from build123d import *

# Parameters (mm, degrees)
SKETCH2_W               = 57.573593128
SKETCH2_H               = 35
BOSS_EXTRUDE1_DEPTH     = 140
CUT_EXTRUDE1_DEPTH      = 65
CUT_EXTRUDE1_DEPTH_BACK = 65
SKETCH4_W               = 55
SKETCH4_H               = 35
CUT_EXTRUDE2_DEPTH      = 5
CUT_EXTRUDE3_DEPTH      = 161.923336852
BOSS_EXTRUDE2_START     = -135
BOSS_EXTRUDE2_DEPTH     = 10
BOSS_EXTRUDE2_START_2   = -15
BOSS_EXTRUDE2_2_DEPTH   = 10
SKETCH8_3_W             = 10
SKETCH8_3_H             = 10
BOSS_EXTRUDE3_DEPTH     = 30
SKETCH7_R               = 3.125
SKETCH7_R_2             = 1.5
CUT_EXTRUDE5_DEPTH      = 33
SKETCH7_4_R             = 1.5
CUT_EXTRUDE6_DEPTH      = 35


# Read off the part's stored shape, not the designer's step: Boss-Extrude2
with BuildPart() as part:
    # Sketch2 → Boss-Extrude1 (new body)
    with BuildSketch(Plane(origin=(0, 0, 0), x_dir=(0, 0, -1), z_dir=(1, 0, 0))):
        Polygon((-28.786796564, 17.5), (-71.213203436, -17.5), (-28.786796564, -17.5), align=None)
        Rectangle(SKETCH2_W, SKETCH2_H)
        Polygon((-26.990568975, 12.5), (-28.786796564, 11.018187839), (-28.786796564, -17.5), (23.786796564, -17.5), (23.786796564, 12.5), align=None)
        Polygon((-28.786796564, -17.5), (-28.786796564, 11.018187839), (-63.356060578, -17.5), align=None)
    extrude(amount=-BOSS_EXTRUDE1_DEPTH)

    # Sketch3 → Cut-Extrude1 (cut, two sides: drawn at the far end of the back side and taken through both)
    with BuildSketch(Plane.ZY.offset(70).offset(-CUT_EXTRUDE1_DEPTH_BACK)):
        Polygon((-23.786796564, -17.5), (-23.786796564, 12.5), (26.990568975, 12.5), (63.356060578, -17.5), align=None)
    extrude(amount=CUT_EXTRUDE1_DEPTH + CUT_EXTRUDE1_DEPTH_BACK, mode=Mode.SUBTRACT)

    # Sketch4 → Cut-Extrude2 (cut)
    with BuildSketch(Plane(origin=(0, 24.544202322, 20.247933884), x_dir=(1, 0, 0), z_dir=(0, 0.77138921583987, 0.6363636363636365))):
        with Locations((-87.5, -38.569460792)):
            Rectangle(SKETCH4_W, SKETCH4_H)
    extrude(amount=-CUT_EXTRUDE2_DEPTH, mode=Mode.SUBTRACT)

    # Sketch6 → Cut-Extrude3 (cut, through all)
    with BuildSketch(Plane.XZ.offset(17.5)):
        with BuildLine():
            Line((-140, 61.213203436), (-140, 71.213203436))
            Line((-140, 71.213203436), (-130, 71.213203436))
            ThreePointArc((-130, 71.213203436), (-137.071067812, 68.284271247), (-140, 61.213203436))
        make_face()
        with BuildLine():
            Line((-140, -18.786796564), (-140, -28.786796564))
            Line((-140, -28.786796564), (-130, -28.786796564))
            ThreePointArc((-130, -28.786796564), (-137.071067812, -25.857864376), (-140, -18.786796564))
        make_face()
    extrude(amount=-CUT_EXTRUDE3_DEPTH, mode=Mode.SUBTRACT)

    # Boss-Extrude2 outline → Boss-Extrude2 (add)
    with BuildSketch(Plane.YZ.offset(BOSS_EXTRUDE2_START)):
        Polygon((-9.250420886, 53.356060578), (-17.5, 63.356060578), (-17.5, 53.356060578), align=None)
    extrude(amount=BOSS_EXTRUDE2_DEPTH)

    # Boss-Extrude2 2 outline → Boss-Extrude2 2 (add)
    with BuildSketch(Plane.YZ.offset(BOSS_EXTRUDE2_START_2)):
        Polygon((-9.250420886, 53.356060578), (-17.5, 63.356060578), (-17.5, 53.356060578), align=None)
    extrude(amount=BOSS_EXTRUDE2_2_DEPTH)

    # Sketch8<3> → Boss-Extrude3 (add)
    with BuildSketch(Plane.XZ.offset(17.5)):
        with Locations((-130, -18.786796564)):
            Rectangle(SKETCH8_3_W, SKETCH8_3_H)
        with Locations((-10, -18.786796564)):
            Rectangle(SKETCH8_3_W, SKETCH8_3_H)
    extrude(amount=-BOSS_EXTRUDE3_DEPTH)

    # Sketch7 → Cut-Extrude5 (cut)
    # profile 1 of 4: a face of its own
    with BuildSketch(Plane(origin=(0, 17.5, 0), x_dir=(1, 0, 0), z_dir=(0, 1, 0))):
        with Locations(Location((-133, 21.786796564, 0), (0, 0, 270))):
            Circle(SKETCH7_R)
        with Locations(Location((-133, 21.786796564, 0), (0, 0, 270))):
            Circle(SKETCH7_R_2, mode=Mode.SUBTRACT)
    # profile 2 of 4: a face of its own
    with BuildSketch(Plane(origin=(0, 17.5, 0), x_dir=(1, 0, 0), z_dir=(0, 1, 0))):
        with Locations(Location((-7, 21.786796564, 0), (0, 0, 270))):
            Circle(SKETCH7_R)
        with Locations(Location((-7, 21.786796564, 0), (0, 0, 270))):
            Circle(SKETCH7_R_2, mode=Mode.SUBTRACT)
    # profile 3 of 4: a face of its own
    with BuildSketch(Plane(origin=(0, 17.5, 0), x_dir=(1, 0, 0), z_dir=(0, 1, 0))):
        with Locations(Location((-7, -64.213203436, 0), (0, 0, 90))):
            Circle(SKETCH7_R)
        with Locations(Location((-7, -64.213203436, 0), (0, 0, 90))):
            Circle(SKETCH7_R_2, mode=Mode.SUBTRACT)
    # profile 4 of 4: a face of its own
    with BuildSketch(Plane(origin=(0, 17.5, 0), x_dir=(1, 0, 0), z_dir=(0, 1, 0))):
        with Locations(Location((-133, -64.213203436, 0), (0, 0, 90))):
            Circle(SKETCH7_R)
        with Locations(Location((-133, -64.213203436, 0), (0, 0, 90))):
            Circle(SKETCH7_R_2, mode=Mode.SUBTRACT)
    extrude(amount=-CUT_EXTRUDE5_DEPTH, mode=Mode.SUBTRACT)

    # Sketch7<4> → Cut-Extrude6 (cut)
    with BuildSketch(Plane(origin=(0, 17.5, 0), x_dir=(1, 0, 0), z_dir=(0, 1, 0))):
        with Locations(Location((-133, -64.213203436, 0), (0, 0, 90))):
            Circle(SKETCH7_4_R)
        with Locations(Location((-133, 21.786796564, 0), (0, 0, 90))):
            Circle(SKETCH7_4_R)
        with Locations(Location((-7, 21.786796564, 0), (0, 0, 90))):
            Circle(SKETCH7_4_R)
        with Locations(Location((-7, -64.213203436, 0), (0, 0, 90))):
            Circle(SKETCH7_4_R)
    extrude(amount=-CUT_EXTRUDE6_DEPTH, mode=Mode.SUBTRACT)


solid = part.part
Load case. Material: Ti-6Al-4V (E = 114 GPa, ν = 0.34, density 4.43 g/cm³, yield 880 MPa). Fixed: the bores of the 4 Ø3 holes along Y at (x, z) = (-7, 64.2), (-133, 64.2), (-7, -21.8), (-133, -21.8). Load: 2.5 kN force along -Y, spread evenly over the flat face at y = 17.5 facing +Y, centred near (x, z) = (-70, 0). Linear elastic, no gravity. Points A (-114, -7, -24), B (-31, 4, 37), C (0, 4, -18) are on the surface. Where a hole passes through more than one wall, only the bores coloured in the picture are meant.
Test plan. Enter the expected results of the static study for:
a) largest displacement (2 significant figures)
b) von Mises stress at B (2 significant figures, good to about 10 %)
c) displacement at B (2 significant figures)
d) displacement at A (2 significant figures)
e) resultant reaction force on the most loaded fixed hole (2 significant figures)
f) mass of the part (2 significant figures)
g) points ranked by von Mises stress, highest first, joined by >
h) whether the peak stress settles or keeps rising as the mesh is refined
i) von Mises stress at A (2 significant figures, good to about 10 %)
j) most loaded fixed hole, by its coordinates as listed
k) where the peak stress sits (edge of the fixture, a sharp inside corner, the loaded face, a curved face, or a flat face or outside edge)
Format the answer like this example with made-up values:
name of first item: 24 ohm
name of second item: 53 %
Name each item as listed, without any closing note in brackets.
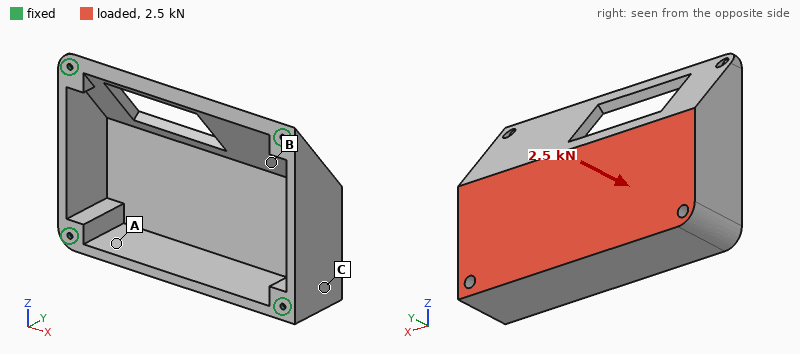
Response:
largest displacement: 32 µm
von Mises stress at B: 7.6 MPa
displacement at B: 11 µm
displacement at A: 8.8 µm
resultant reaction force on the most loaded fixed hole: 1.2 kN
mass of the part: 490 g
points ranked by von Mises stress, highest first, joined by >: A > B > C
whether the peak stress settles or keeps rising as the mesh is refined: keeps rising
von Mises stress at A: 11 MPa
most loaded fixed hole, by its coordinates as listed: (-133, -21.8)
where the peak stress sits: edge of the fixture
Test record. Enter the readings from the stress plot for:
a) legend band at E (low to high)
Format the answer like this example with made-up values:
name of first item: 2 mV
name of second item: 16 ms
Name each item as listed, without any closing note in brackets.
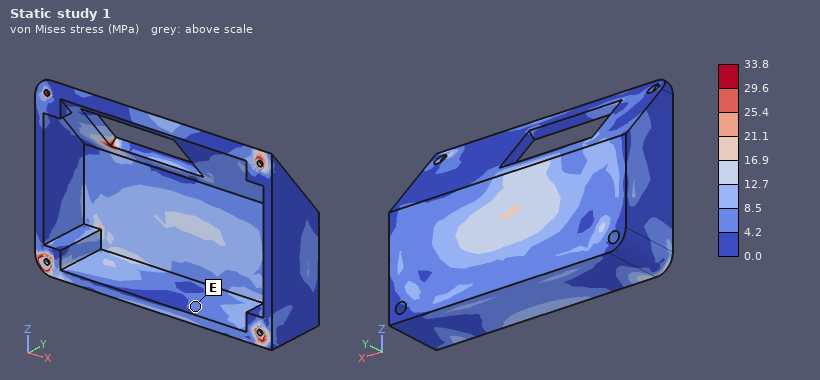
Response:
legend band at E: 4.2 to 8.5 MPa
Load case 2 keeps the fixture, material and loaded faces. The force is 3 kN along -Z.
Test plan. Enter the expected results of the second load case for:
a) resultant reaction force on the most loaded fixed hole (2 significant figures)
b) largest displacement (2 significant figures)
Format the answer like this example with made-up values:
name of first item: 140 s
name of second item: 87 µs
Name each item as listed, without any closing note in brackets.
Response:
resultant reaction force on the most loaded fixed hole: 1.2 kN
largest displacement: 20 µm
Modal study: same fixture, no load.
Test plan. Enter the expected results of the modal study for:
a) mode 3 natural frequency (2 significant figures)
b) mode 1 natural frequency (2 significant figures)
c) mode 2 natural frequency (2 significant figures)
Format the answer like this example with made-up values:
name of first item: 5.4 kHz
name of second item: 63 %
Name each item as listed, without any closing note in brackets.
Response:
mode 3 natural frequency: 3800 Hz
mode 1 natural frequency: 2100 Hz
mode 2 natural frequency: 3000 Hz
